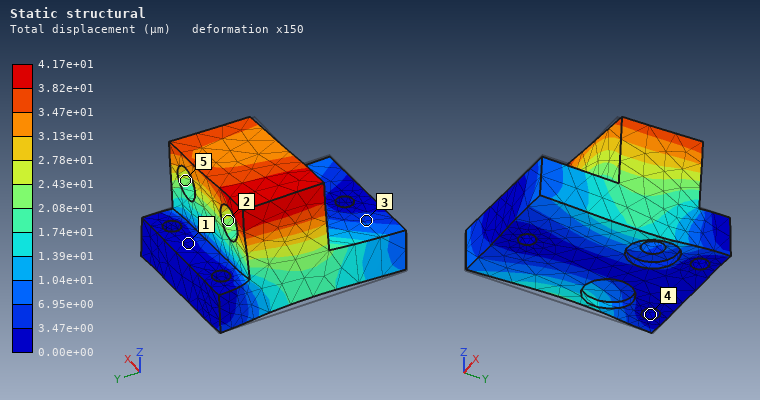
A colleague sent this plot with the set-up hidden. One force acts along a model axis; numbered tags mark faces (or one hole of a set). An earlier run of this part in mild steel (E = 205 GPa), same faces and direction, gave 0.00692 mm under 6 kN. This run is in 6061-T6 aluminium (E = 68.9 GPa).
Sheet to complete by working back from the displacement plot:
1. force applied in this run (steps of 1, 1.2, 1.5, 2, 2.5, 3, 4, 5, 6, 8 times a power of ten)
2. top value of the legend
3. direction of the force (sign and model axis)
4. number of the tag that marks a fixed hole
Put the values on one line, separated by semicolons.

12 kN; 4.17e+01 µm; +X; 4
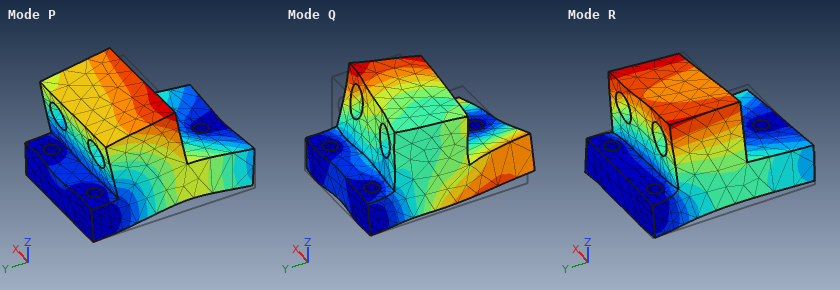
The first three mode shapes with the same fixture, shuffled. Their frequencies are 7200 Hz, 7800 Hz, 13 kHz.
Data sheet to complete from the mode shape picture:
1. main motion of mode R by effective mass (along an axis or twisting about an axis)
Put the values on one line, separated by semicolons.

along X
